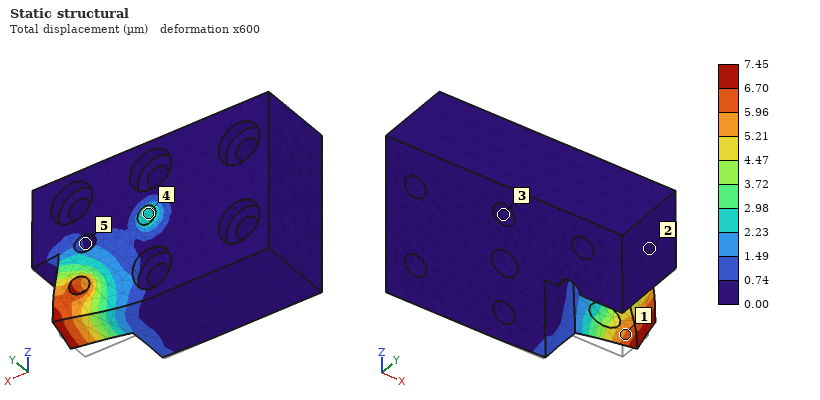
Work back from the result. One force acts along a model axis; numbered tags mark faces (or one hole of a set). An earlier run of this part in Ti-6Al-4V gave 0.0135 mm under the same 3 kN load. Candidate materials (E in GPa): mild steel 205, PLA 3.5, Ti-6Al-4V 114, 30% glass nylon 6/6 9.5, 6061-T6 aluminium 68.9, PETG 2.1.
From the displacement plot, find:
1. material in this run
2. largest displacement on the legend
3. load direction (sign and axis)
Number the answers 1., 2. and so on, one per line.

1. mild steel
2. 7.45 µm
3. +Y
